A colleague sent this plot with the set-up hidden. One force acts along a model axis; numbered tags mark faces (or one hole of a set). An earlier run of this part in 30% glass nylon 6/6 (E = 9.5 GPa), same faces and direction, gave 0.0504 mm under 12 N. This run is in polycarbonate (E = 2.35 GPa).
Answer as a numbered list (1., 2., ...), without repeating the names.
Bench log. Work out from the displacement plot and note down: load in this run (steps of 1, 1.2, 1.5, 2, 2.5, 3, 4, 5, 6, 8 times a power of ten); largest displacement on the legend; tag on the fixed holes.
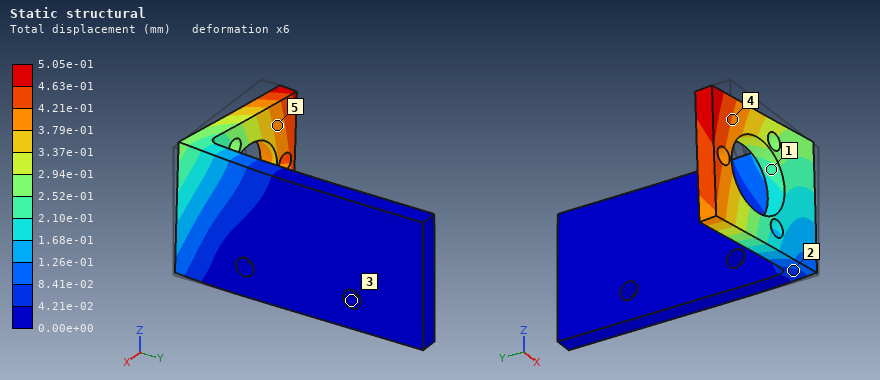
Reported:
1. 30 N
2. 5.05e-01 mm
3. 3
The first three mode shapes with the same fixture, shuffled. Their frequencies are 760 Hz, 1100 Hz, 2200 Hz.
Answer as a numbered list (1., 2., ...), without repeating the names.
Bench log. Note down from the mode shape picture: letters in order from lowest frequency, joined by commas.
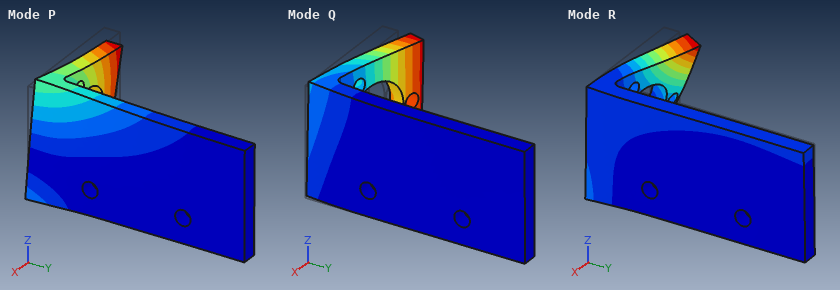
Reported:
1. Q, P, R
